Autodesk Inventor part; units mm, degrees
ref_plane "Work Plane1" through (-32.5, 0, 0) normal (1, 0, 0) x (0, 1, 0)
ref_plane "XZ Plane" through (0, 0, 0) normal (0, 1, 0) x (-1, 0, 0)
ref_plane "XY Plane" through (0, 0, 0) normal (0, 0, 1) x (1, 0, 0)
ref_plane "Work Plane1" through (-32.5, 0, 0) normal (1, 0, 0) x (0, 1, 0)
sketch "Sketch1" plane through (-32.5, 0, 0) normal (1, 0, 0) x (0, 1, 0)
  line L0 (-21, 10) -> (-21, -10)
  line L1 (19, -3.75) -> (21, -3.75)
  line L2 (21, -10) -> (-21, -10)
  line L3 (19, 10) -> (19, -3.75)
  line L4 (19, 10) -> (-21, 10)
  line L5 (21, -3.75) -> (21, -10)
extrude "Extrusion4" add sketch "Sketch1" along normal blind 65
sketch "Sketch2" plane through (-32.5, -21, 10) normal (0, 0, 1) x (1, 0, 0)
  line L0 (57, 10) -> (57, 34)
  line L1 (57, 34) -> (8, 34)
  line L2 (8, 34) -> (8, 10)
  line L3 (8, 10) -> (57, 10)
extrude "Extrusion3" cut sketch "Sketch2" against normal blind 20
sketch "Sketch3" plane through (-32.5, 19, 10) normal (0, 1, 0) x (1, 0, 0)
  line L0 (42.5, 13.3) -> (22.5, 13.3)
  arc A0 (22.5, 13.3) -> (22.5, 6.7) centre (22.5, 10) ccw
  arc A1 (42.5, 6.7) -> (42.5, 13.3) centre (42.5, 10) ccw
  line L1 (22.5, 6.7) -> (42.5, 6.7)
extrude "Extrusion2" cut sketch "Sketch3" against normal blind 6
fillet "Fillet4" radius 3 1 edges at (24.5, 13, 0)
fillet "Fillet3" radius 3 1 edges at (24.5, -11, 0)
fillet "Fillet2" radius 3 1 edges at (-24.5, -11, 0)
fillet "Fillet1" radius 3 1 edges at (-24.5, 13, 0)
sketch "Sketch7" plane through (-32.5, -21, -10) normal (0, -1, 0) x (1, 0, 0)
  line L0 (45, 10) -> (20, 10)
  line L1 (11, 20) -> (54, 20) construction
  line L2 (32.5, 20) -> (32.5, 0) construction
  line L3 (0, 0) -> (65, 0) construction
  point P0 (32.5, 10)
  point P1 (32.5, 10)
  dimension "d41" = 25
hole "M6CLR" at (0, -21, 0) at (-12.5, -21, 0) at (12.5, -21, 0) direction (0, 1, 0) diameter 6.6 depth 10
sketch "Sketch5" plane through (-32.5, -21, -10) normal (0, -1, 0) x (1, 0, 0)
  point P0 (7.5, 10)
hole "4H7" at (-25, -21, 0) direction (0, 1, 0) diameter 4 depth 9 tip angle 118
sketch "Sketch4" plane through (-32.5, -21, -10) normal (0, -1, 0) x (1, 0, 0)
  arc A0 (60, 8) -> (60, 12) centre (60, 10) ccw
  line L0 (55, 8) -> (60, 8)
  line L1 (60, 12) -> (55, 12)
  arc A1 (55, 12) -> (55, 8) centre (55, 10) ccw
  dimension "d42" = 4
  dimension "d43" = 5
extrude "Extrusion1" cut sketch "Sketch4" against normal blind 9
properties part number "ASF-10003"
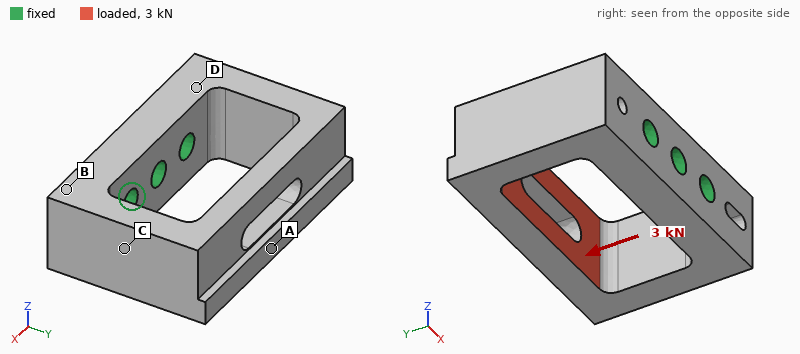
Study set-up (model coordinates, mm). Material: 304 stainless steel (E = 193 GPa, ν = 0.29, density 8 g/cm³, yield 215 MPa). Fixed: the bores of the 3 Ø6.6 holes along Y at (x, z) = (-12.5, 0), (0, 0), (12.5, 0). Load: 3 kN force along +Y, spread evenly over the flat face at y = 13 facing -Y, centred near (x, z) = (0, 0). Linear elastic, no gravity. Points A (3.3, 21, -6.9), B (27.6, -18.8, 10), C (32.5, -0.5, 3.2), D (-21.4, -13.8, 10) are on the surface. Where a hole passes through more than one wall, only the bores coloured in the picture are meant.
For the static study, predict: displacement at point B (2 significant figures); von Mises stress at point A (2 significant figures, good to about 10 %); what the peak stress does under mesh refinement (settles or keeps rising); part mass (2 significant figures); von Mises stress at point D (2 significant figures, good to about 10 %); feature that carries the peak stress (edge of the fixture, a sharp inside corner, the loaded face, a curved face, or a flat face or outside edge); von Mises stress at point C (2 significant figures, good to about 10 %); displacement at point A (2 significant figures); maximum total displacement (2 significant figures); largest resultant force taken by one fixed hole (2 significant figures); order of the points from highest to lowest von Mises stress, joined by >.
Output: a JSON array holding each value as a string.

["6.3 µm", "82 MPa", "keeps rising", "220 g", "18 MPa", "edge of the fixture", "29 MPa", "34 µm", "42 µm", "1.8 kN", "A > C > D > B"]
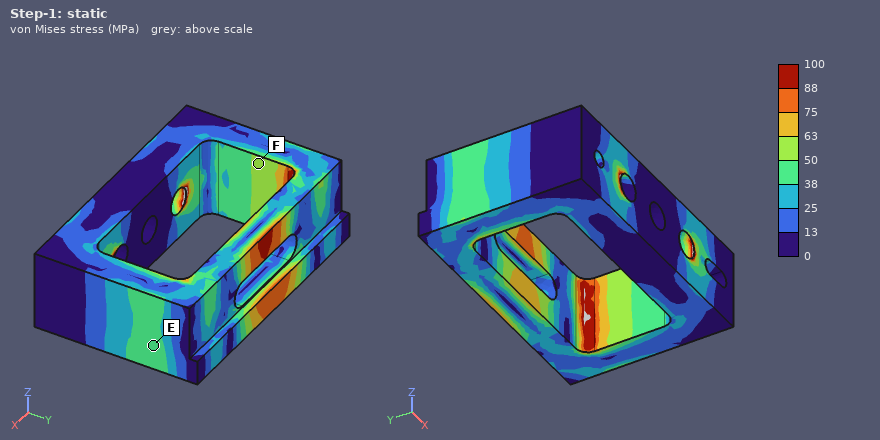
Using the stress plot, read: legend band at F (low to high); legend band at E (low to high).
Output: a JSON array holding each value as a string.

["50 to 63 MPa", "38 to 50 MPa"]
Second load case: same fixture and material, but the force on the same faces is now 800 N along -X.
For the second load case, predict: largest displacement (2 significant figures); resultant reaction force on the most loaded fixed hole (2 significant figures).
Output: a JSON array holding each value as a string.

["23 µm", "460 N"]
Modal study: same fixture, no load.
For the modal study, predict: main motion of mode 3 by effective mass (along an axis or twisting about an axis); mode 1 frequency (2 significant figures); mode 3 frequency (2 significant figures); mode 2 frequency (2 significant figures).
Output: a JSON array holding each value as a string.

["twisting about Y", "3400 Hz", "5200 Hz", "3400 Hz"]
